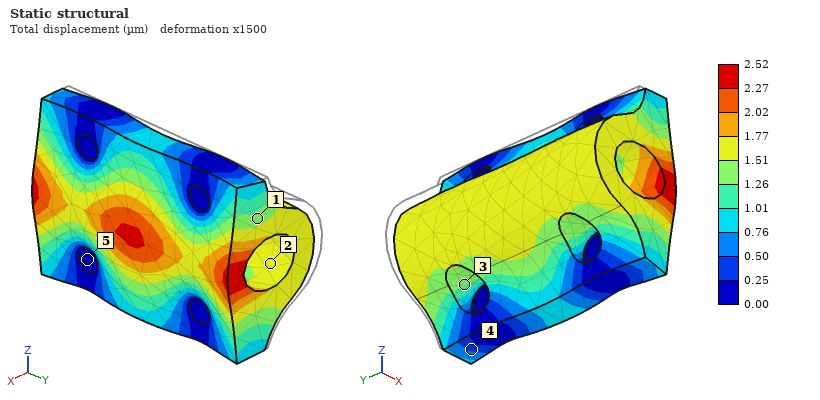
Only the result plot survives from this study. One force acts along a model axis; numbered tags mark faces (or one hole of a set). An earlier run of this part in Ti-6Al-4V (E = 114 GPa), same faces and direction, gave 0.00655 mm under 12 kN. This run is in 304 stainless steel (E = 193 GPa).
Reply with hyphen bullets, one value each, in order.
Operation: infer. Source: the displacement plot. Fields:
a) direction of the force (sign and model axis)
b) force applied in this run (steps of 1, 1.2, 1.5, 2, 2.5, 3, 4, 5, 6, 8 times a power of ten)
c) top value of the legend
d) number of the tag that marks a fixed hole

- +X
- 8 kN
- 2.52 µm
- 5
